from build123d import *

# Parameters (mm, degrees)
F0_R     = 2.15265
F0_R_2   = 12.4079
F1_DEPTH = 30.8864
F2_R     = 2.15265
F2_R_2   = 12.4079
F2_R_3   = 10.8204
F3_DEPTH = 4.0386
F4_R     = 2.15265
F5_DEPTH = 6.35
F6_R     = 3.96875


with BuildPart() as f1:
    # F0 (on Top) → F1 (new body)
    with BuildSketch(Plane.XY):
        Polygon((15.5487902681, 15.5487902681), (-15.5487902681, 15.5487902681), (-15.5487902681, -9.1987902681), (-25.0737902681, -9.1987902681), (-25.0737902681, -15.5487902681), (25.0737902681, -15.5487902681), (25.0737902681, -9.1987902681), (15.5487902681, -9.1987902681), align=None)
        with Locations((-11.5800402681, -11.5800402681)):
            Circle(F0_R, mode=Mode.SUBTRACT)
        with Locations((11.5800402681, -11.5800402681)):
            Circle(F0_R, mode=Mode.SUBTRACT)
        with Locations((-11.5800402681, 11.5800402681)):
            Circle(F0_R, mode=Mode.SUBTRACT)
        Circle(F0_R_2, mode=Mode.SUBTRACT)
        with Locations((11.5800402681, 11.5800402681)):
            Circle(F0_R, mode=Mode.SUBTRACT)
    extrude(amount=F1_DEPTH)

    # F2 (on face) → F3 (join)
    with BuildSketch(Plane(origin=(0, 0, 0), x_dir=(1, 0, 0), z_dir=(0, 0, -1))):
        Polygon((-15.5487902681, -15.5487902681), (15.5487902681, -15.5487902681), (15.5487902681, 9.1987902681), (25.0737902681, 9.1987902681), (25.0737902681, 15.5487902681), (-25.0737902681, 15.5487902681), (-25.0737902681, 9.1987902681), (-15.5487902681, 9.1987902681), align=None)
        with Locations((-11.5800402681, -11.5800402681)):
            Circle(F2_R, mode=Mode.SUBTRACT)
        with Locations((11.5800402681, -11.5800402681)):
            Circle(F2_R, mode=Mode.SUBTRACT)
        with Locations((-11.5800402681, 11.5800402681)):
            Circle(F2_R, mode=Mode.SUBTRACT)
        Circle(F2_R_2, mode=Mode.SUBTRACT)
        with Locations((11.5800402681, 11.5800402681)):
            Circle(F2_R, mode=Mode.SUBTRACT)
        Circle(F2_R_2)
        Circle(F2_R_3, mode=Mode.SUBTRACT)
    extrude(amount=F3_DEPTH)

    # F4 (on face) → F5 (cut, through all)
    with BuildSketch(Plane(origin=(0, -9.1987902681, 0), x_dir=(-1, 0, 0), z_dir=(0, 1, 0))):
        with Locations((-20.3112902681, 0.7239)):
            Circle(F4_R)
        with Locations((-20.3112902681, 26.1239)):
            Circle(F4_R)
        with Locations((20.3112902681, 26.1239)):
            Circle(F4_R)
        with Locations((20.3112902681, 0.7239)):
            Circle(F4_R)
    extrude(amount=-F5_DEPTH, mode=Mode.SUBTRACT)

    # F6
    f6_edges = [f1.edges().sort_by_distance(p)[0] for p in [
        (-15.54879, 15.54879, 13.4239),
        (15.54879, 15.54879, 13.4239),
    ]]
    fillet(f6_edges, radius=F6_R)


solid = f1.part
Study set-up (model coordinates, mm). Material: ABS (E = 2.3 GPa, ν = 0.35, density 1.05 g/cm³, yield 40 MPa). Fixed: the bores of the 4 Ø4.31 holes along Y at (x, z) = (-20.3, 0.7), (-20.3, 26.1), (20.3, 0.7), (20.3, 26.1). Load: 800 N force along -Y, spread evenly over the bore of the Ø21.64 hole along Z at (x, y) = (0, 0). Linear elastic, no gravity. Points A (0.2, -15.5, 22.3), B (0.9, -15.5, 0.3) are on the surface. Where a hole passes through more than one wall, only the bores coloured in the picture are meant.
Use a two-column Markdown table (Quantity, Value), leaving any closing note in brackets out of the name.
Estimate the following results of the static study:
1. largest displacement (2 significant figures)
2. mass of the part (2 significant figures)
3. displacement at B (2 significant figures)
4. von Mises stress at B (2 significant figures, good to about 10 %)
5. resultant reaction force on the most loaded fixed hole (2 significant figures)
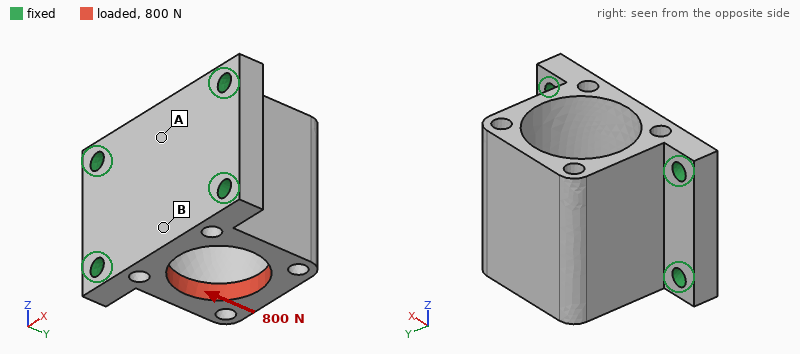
| Quantity | Value |
|---|---|
| largest displacement | 0.24 mm |
| mass of the part | 20 g |
| displacement at B | 0.19 mm |
| von Mises stress at B | 9.3 MPa |
| resultant reaction force on the most loaded fixed hole | 430 N |
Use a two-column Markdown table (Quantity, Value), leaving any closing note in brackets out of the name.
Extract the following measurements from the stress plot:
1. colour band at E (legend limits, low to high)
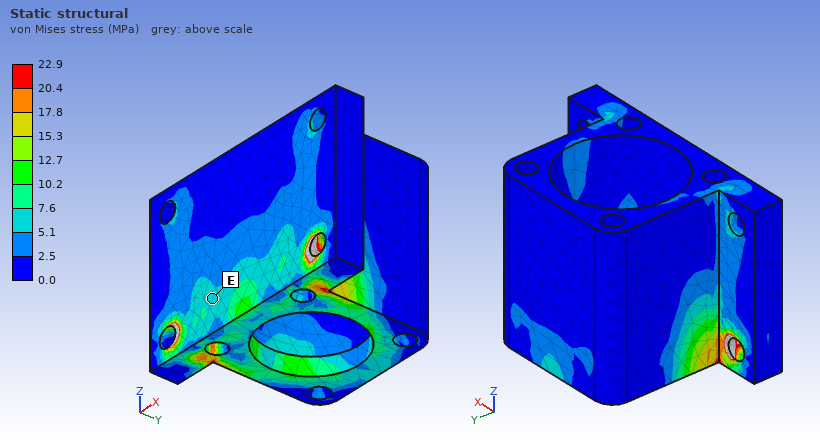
| Quantity | Value |
|---|---|
| colour band at E | 5.1 to 7.6 MPa |
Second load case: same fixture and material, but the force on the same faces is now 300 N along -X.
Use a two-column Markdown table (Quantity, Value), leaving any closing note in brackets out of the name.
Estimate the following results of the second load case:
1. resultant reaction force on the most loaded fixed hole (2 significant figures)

| Quantity | Value |
|---|---|
| resultant reaction force on the most loaded fixed hole | 110 N |
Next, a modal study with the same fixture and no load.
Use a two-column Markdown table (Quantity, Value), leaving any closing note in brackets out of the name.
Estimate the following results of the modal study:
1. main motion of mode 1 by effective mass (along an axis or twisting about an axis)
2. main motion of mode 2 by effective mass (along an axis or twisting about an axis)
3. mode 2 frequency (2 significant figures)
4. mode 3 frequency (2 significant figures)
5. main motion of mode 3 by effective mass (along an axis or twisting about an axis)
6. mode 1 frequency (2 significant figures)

| Quantity | Value |
|---|---|
| main motion of mode 1 by effective mass | along X |
| main motion of mode 2 by effective mass | along Z |
| mode 2 frequency | 3100 Hz |
| mode 3 frequency | 3900 Hz |
| main motion of mode 3 by effective mass | twisting about Y |
| mode 1 frequency | 2100 Hz |
